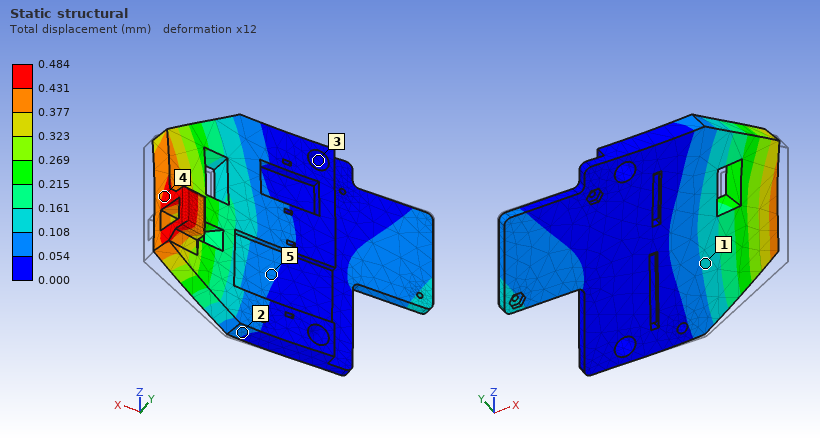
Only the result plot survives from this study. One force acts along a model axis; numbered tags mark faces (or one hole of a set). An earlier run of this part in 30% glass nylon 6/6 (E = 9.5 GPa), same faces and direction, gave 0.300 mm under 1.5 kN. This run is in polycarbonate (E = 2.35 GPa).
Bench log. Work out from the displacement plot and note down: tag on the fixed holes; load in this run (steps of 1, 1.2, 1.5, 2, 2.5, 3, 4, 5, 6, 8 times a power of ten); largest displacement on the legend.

3
600 N
0.484 mm
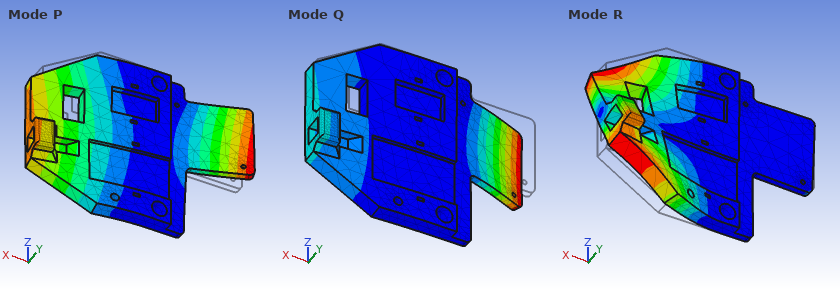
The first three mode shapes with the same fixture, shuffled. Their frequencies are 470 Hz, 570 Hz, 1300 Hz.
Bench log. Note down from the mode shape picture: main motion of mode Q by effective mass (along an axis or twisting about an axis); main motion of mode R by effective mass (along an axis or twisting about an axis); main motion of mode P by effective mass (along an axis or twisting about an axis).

along Y
twisting about X
along Y
